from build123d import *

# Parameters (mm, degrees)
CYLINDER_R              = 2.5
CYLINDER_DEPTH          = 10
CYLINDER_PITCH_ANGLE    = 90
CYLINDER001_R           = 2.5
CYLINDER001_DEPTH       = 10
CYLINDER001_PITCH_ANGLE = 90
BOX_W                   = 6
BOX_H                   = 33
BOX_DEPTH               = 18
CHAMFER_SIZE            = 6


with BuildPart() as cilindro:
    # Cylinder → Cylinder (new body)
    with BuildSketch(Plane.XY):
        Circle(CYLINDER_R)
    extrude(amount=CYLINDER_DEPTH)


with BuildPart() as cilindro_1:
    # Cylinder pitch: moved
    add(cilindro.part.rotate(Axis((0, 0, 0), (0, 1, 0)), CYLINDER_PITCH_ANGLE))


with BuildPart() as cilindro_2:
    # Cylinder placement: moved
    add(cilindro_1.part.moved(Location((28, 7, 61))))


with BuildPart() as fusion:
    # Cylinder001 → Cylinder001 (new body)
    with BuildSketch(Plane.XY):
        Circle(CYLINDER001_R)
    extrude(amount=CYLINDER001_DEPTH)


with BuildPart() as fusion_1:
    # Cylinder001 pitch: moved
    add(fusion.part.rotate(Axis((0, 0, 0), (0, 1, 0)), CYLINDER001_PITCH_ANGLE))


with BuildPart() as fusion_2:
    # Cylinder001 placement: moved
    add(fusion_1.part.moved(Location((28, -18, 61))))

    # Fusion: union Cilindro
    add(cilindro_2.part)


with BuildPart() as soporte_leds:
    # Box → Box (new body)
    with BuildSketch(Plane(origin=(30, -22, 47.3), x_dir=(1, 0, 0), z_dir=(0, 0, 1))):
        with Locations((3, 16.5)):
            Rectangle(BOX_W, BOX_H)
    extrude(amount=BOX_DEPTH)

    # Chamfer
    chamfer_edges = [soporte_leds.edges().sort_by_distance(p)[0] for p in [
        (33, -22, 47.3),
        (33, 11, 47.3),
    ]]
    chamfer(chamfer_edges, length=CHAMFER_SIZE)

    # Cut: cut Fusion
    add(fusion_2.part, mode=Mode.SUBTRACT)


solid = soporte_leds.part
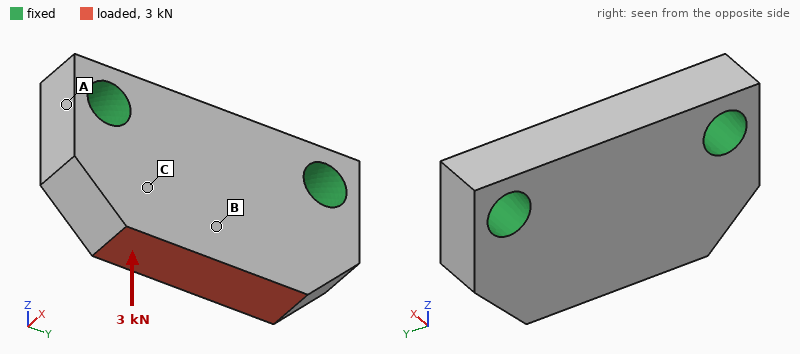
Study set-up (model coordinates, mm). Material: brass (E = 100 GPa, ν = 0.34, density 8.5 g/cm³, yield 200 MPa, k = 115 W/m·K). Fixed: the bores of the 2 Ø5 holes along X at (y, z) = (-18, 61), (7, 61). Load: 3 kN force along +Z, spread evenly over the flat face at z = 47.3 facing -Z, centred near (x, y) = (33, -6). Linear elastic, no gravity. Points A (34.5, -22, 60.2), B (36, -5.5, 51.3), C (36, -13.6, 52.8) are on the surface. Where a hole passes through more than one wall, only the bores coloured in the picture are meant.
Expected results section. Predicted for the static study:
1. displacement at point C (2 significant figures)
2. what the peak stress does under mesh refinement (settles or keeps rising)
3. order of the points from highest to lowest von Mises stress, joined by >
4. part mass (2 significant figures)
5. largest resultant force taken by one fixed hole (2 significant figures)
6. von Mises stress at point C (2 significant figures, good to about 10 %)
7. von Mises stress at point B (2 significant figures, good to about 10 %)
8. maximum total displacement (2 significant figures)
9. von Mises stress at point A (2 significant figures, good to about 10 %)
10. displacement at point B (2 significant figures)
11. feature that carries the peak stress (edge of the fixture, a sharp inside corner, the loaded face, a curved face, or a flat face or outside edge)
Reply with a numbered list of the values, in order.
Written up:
1. 2.5 µm
2. keeps rising
3. C > B > A
4. 26 g
5. 1.6 kN
6. 27 MPa
7. 19 MPa
8. 5.0 µm
9. 7.1 MPa
10. 4.3 µm
11. edge of the fixture
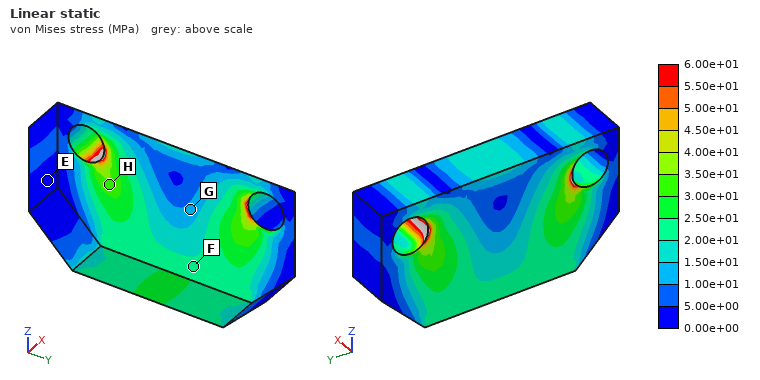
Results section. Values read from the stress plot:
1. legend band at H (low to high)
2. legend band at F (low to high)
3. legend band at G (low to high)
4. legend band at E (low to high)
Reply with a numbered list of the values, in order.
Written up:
1. 3.00e+01 to 3.50e+01 MPa
2. 2.00e+01 to 2.50e+01 MPa
3. 1.00e+01 to 1.50e+01 MPa
4. 0.00e+00 to 5.00e+00 MPa
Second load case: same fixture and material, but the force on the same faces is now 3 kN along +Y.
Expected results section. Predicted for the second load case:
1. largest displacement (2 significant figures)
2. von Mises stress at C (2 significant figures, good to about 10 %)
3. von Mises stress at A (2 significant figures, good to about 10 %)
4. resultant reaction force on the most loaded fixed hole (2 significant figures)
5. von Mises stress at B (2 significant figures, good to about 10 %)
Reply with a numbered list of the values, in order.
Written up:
1. 7.6 µm
2. 31 MPa
3. 32 MPa
4. 2.1 kN
5. 38 MPa
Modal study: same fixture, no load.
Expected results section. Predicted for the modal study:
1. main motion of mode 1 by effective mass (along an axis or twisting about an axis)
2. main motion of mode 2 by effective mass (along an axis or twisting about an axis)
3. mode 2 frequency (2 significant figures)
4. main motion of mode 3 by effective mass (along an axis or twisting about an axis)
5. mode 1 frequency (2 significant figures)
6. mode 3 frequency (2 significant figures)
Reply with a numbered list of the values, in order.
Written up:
1. along X
2. twisting about Z
3. 29 kHz
4. along X
5. 15 kHz
6. 32 kHz
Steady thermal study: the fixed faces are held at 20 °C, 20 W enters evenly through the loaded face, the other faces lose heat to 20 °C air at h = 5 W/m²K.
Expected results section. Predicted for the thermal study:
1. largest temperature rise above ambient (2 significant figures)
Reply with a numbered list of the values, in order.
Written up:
1. 17 K
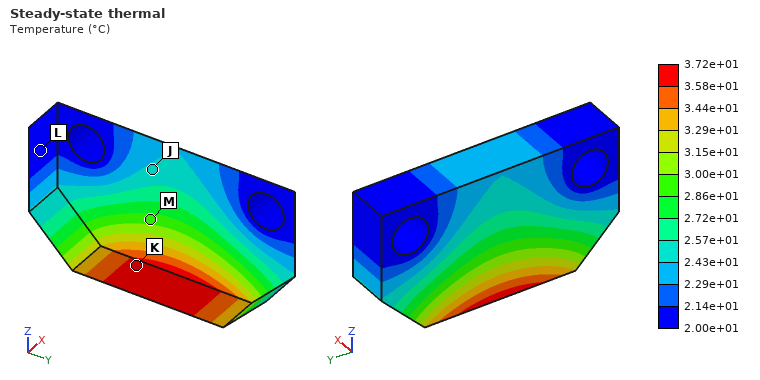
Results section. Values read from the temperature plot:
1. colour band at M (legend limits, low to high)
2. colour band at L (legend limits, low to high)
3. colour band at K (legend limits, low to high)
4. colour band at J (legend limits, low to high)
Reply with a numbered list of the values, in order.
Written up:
1. 2.86e+01 to 3.00e+01 °C
2. 2.00e+01 to 2.14e+01 °C
3. 3.58e+01 to 3.72e+01 °C
4. 2.43e+01 to 2.57e+01 °C
